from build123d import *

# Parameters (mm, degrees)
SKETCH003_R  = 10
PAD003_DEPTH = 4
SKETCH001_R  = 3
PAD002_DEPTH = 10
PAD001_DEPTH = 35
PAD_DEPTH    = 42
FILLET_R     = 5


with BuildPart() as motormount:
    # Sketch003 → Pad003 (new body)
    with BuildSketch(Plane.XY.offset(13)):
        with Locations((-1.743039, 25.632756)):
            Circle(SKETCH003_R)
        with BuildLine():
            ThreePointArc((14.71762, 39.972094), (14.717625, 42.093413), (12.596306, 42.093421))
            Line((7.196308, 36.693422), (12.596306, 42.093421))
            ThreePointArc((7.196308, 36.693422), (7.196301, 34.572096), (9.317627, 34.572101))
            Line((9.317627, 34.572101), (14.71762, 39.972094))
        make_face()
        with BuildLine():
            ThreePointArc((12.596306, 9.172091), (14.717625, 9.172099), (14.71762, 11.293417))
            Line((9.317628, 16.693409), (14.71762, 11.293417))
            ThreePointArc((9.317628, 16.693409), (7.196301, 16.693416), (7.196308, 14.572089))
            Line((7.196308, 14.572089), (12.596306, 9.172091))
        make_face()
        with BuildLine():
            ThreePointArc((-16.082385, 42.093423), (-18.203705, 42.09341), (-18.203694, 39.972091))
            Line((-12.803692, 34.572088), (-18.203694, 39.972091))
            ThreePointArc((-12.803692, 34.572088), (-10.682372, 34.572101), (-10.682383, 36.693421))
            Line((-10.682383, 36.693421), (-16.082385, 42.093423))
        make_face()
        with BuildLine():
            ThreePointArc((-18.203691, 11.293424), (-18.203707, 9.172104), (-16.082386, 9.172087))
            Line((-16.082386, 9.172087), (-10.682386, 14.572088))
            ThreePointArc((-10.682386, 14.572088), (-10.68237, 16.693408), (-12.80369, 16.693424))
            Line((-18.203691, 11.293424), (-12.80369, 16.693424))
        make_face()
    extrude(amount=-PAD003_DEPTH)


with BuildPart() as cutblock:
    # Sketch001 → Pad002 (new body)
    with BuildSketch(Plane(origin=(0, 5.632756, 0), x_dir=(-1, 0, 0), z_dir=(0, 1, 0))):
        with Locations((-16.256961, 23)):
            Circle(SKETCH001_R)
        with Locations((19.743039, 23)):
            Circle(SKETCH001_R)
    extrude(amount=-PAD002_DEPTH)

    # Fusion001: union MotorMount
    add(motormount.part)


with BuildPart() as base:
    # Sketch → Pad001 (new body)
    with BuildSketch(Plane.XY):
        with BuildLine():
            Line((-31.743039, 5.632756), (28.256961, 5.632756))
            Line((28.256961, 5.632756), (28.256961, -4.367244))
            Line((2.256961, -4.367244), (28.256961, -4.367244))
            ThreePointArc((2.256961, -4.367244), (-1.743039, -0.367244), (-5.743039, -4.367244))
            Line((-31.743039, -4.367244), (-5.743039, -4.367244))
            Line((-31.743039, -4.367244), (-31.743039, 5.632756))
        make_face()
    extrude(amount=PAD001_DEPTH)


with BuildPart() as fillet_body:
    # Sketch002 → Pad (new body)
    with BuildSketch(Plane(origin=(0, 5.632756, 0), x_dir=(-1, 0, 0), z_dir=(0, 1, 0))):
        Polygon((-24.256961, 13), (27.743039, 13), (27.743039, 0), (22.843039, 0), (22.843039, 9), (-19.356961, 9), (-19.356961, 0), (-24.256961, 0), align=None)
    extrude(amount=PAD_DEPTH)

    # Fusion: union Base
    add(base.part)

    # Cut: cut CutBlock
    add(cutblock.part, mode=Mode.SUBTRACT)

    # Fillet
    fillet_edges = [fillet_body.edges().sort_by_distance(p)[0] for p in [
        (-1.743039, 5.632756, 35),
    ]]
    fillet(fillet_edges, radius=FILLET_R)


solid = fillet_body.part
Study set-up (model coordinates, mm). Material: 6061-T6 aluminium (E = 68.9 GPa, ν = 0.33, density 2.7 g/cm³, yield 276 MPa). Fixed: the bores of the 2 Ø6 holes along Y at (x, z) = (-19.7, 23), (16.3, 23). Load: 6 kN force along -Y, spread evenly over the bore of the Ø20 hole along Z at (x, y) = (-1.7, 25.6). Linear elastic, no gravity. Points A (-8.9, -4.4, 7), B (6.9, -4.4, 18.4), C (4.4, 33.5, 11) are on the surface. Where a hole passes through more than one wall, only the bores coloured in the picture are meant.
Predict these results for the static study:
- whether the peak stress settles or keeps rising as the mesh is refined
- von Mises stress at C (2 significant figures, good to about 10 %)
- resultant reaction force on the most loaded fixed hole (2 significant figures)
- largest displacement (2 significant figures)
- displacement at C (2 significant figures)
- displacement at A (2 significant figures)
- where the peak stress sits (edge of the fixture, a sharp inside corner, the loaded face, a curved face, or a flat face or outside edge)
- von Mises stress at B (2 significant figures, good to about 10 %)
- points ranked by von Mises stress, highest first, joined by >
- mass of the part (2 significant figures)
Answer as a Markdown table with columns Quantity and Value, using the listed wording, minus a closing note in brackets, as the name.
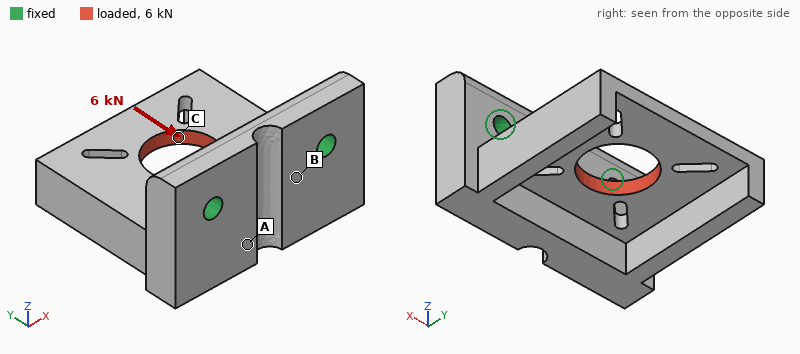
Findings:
| Quantity | Value |
|---|---|
| whether the peak stress settles or keeps rising as the mesh is refined | keeps rising |
| von Mises stress at C | 39 MPa |
| resultant reaction force on the most loaded fixed hole | 3.0 kN |
| largest displacement | 67 µm |
| displacement at C | 60 µm |
| displacement at A | 27 µm |
| where the peak stress sits | edge of the fixture |
| von Mises stress at B | 23 MPa |
| points ranked by von Mises stress, highest first, joined by > | C > B > A |
| mass of the part | 81 g |
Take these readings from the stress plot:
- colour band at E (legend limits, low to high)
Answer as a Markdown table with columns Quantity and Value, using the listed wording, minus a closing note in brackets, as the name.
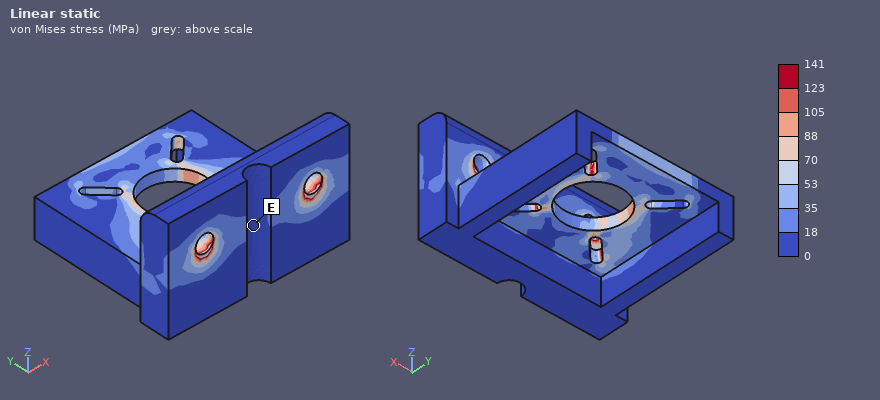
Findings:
| Quantity | Value |
|---|---|
| colour band at E | 0 to 18 MPa |
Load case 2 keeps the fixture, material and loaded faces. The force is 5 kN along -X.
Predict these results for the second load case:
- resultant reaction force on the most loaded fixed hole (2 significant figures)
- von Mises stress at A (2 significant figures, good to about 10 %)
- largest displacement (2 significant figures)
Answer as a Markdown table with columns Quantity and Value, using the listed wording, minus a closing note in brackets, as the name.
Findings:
| Quantity | Value |
|---|---|
| resultant reaction force on the most loaded fixed hole | 4.1 kN |
| von Mises stress at A | 15 MPa |
| largest displacement | 0.12 mm |
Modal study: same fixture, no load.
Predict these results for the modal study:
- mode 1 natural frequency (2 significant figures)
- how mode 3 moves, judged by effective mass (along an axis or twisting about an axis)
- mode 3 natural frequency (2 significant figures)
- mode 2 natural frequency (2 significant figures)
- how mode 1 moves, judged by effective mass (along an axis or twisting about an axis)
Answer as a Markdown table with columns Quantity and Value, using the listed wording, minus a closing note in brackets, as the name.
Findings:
| Quantity | Value |
|---|---|
| mode 1 natural frequency | 2900 Hz |
| how mode 3 moves, judged by effective mass | along X |
| mode 3 natural frequency | 6400 Hz |
| mode 2 natural frequency | 4100 Hz |
| how mode 1 moves, judged by effective mass | along Z |
